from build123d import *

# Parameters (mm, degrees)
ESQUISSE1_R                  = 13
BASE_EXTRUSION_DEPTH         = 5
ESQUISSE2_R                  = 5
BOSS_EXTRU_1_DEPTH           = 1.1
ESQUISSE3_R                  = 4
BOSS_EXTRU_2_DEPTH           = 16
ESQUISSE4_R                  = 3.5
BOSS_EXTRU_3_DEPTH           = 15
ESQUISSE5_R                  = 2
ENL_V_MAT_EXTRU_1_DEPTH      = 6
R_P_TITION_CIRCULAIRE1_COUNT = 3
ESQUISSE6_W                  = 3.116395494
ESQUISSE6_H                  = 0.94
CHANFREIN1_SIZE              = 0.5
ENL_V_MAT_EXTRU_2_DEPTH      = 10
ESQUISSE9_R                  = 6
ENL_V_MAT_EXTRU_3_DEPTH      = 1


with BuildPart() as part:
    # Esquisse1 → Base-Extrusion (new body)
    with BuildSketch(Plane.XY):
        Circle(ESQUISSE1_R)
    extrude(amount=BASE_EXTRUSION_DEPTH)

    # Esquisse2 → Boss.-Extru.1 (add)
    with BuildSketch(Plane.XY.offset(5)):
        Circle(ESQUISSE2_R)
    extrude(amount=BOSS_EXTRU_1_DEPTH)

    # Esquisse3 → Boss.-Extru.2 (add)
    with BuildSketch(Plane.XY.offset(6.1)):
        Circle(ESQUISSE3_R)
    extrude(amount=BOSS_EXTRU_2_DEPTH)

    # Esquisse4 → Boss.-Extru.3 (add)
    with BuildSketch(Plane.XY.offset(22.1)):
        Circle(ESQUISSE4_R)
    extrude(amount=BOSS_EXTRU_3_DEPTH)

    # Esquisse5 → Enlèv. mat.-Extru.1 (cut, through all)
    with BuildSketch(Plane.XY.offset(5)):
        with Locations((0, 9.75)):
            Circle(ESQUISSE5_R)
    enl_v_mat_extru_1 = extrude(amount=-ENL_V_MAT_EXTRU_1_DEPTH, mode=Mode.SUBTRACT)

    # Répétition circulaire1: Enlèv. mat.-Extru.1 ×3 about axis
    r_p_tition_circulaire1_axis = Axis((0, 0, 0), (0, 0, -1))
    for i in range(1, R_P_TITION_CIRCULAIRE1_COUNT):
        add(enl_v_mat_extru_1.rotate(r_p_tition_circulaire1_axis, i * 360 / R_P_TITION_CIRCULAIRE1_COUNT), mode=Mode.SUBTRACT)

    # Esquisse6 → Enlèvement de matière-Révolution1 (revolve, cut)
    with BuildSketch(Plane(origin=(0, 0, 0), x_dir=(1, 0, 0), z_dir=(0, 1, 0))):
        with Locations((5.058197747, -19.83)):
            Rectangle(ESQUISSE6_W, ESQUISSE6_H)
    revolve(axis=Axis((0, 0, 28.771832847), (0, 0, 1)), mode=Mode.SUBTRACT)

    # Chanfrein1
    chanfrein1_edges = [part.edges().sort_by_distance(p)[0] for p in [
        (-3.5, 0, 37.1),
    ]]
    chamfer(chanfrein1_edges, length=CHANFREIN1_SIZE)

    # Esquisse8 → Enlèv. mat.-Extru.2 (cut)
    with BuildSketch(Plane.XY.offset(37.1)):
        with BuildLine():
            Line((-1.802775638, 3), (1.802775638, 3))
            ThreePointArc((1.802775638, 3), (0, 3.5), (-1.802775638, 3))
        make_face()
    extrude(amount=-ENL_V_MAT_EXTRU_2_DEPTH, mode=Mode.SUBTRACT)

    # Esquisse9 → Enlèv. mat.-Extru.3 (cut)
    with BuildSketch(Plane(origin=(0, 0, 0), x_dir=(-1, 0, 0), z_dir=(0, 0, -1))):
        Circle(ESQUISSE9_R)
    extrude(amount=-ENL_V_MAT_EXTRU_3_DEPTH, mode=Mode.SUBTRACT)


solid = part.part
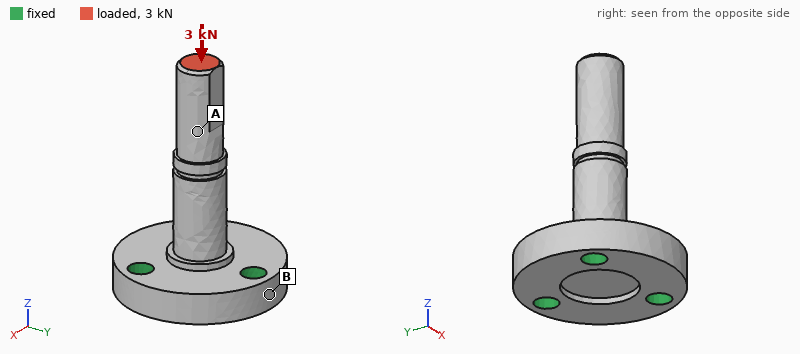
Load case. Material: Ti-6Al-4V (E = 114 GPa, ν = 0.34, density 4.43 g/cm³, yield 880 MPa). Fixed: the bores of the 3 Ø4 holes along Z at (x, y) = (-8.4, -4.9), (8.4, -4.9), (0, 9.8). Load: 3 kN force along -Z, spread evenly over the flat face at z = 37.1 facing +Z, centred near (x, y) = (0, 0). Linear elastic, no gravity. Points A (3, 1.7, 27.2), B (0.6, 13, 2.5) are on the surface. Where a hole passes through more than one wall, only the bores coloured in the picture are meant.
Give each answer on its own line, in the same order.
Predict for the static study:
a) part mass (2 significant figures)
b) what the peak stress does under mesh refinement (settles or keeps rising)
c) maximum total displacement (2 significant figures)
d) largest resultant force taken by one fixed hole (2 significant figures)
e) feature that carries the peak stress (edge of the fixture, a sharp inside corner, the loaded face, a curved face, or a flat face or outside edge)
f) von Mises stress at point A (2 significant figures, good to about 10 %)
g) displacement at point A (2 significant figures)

17 g
keeps rising
26 µm
1.1 kN
edge of the fixture
81 MPa
17 µm
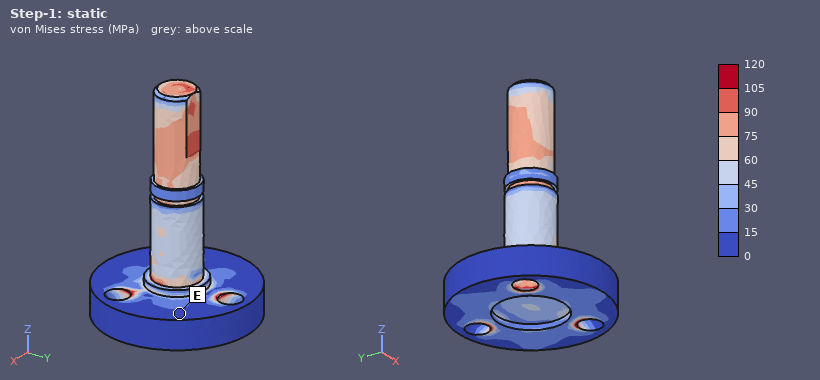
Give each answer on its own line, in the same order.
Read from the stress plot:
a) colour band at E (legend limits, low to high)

0 to 15 MPa
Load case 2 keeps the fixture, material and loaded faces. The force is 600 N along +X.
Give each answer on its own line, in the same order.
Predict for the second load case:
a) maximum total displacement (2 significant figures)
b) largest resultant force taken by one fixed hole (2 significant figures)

0.38 mm
1.3 kN
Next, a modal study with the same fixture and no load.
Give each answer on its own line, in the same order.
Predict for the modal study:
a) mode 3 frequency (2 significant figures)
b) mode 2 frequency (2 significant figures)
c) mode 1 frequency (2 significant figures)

25 kHz
5500 Hz
5500 Hz
